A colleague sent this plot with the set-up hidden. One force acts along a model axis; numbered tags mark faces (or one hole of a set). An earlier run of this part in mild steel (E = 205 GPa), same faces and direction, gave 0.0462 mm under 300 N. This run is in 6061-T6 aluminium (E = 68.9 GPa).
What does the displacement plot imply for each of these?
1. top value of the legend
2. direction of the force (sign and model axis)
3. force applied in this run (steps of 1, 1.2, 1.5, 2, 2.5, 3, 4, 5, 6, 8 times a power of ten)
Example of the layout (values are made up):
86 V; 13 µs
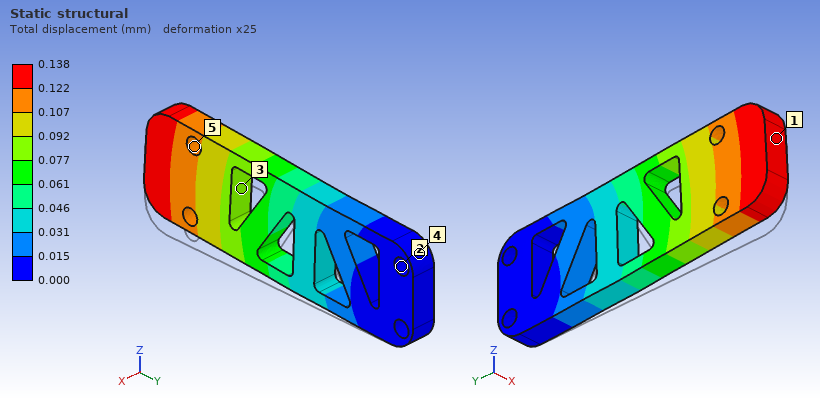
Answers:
0.138 mm; +Z; 300 N
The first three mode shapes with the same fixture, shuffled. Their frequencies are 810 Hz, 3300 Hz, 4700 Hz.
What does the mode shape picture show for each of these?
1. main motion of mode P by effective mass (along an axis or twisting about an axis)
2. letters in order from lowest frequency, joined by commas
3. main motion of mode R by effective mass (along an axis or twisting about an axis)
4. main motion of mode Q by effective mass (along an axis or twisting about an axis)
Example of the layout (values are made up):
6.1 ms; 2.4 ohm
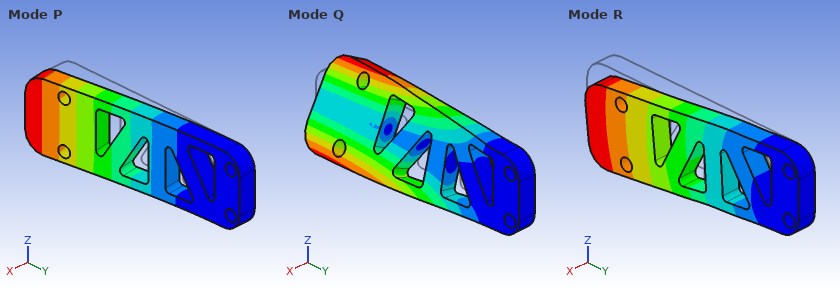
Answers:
along X; P, R, Q; along Z; twisting about Y
